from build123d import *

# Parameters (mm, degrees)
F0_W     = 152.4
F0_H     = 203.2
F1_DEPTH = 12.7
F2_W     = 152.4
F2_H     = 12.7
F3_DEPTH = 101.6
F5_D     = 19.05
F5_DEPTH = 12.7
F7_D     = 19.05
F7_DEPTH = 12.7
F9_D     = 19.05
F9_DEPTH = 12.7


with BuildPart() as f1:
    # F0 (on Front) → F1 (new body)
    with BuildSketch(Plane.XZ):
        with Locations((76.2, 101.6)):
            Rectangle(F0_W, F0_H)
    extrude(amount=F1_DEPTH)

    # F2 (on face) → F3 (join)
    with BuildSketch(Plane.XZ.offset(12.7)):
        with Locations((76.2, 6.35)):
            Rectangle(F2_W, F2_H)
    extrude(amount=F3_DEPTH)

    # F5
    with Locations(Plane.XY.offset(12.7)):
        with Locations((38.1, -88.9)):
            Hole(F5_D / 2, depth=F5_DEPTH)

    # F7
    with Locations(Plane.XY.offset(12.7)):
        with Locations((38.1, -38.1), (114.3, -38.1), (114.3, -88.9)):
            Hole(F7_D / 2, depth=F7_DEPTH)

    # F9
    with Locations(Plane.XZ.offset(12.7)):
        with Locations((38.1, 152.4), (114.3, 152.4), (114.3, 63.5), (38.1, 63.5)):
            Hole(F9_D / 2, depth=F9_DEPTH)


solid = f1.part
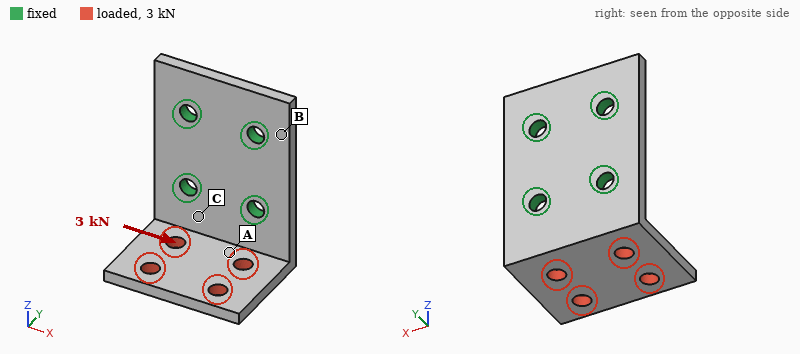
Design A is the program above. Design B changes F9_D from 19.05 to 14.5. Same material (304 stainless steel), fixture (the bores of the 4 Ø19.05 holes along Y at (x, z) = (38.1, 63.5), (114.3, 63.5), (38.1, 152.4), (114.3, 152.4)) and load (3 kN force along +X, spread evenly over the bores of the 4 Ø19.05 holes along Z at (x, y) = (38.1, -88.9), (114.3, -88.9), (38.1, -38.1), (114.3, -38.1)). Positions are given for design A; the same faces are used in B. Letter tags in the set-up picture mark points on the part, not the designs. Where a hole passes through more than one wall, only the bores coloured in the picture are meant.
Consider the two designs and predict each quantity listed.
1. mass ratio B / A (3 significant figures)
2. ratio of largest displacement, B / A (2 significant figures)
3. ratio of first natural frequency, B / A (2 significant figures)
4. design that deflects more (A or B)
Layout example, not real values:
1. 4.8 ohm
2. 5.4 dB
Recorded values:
1. 1.01
2. 1.1
3. 0.97
4. B
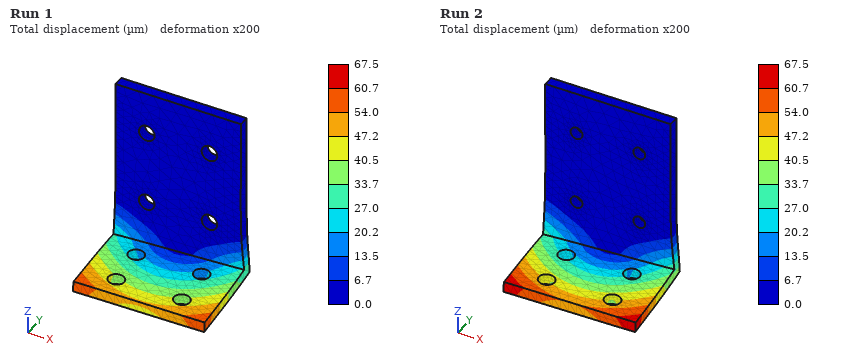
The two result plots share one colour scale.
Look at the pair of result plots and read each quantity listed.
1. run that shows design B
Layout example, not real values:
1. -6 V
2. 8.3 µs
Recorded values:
1. Run 2
